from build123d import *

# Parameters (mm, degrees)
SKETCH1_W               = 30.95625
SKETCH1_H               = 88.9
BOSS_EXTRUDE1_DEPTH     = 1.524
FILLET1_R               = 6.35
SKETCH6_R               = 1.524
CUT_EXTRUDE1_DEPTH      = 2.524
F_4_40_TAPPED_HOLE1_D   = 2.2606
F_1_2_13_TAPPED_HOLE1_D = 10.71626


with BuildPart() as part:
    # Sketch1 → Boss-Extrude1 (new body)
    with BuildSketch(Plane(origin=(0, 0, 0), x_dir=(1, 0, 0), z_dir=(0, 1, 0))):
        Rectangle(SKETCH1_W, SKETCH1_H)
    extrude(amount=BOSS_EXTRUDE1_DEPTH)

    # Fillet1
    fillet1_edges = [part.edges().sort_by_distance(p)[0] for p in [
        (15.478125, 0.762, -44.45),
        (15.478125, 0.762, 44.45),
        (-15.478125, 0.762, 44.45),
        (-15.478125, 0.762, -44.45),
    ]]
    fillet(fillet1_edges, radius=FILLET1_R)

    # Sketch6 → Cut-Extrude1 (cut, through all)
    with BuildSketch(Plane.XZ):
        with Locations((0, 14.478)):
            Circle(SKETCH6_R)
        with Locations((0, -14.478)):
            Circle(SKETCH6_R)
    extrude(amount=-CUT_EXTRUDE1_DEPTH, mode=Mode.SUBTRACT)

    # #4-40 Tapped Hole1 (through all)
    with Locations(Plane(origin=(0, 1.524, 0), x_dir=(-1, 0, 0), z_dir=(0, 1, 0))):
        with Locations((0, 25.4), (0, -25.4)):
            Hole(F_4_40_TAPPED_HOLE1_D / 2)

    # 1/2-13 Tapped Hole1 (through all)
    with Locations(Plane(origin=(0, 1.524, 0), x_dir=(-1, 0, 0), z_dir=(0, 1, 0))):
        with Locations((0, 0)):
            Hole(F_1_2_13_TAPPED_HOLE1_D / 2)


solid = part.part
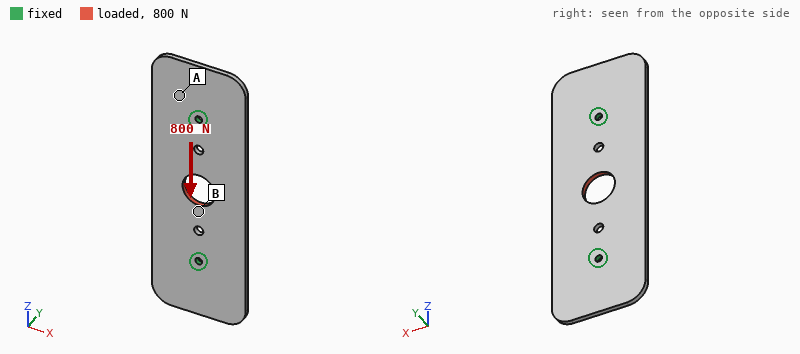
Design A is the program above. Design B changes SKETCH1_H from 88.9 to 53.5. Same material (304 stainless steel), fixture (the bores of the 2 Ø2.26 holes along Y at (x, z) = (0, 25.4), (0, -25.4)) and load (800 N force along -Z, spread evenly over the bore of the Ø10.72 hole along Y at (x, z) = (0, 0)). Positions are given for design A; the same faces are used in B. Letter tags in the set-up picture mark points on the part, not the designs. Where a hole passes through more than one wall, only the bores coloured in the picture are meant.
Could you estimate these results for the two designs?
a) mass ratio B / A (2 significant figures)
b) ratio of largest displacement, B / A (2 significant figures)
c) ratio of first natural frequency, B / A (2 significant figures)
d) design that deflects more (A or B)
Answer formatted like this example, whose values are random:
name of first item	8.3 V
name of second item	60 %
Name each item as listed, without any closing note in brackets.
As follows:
mass ratio B / A	0.58
ratio of largest displacement, B / A	1.3
ratio of first natural frequency, B / A	0.96
design that deflects more	B
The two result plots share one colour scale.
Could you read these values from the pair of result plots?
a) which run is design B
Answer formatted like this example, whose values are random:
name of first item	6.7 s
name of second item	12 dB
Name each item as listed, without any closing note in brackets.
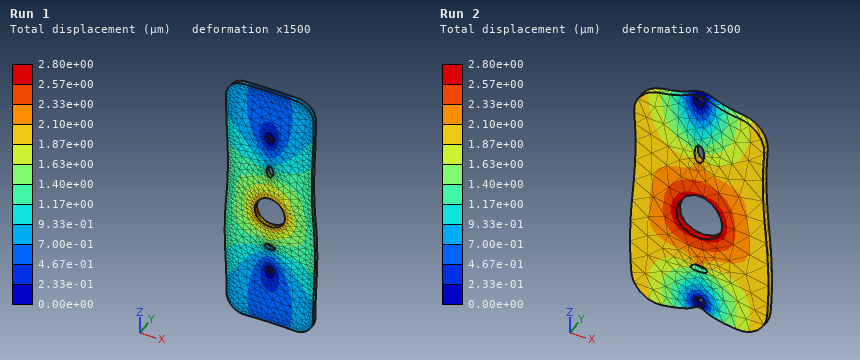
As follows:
which run is design B	Run 2
